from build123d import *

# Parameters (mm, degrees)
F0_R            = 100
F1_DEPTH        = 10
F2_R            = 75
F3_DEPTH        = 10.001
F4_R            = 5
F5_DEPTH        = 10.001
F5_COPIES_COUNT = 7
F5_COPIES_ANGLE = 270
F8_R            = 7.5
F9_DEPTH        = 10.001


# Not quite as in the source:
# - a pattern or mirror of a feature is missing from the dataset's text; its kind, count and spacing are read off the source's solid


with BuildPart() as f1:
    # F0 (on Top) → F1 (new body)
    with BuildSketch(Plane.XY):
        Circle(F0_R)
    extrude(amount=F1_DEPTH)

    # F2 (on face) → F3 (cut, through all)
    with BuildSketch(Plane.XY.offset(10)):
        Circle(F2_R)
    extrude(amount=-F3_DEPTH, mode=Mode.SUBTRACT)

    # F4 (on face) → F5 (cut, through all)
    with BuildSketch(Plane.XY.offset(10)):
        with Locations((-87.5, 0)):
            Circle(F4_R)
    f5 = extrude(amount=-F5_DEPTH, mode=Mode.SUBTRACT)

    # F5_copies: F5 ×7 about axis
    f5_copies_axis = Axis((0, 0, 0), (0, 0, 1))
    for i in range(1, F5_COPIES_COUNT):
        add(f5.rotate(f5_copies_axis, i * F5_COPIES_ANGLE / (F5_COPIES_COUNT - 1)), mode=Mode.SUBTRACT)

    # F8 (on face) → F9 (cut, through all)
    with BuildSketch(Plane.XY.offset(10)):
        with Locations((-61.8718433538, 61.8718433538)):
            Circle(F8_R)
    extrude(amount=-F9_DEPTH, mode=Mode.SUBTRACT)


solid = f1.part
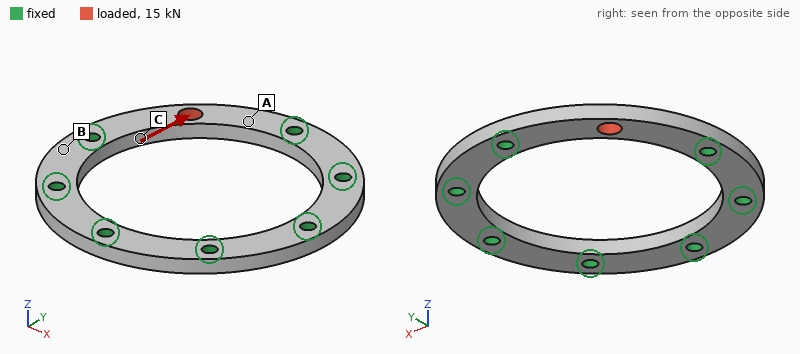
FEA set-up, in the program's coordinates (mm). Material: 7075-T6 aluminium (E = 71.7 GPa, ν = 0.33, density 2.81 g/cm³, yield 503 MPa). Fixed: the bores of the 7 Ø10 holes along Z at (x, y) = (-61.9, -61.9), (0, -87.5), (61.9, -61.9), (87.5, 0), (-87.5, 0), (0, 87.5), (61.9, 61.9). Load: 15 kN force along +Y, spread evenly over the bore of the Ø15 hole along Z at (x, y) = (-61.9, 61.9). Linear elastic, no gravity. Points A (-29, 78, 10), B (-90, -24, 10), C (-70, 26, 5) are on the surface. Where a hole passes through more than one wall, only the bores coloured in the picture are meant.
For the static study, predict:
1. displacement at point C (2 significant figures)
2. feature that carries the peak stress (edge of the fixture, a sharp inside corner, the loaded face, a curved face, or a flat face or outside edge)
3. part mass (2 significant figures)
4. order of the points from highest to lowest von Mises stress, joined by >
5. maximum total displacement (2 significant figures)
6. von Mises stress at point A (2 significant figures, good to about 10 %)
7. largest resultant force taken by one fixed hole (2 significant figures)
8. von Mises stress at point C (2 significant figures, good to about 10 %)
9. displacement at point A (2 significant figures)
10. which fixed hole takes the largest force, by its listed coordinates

0.040 mm
the loaded face
370 g
C > A > B
0.13 mm
32 MPa
14 kN
110 MPa
0.055 mm
(-87.5, 0)
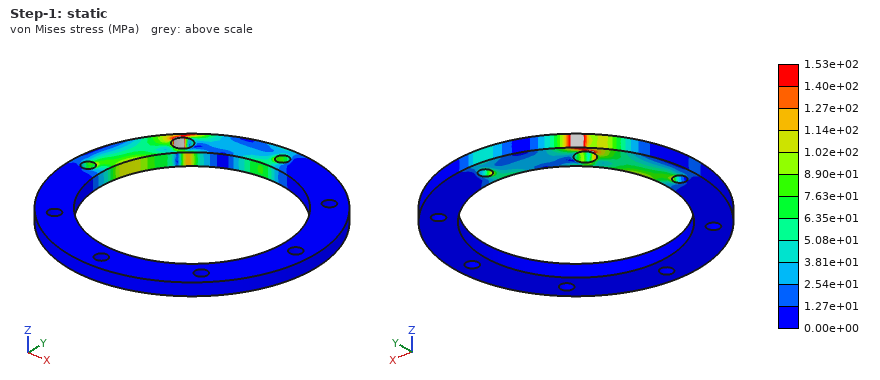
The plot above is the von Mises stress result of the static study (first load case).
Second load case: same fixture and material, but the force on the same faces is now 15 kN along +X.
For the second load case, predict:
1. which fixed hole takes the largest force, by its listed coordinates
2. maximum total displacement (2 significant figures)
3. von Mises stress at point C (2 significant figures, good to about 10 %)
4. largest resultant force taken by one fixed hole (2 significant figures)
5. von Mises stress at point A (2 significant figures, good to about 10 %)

(0, 87.5)
0.13 mm
28 MPa
14 kN
65 MPa
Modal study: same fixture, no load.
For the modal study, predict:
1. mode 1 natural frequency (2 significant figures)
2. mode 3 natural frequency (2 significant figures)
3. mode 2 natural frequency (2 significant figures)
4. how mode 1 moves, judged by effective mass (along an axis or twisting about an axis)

2700 Hz
8700 Hz
6900 Hz
along Z
